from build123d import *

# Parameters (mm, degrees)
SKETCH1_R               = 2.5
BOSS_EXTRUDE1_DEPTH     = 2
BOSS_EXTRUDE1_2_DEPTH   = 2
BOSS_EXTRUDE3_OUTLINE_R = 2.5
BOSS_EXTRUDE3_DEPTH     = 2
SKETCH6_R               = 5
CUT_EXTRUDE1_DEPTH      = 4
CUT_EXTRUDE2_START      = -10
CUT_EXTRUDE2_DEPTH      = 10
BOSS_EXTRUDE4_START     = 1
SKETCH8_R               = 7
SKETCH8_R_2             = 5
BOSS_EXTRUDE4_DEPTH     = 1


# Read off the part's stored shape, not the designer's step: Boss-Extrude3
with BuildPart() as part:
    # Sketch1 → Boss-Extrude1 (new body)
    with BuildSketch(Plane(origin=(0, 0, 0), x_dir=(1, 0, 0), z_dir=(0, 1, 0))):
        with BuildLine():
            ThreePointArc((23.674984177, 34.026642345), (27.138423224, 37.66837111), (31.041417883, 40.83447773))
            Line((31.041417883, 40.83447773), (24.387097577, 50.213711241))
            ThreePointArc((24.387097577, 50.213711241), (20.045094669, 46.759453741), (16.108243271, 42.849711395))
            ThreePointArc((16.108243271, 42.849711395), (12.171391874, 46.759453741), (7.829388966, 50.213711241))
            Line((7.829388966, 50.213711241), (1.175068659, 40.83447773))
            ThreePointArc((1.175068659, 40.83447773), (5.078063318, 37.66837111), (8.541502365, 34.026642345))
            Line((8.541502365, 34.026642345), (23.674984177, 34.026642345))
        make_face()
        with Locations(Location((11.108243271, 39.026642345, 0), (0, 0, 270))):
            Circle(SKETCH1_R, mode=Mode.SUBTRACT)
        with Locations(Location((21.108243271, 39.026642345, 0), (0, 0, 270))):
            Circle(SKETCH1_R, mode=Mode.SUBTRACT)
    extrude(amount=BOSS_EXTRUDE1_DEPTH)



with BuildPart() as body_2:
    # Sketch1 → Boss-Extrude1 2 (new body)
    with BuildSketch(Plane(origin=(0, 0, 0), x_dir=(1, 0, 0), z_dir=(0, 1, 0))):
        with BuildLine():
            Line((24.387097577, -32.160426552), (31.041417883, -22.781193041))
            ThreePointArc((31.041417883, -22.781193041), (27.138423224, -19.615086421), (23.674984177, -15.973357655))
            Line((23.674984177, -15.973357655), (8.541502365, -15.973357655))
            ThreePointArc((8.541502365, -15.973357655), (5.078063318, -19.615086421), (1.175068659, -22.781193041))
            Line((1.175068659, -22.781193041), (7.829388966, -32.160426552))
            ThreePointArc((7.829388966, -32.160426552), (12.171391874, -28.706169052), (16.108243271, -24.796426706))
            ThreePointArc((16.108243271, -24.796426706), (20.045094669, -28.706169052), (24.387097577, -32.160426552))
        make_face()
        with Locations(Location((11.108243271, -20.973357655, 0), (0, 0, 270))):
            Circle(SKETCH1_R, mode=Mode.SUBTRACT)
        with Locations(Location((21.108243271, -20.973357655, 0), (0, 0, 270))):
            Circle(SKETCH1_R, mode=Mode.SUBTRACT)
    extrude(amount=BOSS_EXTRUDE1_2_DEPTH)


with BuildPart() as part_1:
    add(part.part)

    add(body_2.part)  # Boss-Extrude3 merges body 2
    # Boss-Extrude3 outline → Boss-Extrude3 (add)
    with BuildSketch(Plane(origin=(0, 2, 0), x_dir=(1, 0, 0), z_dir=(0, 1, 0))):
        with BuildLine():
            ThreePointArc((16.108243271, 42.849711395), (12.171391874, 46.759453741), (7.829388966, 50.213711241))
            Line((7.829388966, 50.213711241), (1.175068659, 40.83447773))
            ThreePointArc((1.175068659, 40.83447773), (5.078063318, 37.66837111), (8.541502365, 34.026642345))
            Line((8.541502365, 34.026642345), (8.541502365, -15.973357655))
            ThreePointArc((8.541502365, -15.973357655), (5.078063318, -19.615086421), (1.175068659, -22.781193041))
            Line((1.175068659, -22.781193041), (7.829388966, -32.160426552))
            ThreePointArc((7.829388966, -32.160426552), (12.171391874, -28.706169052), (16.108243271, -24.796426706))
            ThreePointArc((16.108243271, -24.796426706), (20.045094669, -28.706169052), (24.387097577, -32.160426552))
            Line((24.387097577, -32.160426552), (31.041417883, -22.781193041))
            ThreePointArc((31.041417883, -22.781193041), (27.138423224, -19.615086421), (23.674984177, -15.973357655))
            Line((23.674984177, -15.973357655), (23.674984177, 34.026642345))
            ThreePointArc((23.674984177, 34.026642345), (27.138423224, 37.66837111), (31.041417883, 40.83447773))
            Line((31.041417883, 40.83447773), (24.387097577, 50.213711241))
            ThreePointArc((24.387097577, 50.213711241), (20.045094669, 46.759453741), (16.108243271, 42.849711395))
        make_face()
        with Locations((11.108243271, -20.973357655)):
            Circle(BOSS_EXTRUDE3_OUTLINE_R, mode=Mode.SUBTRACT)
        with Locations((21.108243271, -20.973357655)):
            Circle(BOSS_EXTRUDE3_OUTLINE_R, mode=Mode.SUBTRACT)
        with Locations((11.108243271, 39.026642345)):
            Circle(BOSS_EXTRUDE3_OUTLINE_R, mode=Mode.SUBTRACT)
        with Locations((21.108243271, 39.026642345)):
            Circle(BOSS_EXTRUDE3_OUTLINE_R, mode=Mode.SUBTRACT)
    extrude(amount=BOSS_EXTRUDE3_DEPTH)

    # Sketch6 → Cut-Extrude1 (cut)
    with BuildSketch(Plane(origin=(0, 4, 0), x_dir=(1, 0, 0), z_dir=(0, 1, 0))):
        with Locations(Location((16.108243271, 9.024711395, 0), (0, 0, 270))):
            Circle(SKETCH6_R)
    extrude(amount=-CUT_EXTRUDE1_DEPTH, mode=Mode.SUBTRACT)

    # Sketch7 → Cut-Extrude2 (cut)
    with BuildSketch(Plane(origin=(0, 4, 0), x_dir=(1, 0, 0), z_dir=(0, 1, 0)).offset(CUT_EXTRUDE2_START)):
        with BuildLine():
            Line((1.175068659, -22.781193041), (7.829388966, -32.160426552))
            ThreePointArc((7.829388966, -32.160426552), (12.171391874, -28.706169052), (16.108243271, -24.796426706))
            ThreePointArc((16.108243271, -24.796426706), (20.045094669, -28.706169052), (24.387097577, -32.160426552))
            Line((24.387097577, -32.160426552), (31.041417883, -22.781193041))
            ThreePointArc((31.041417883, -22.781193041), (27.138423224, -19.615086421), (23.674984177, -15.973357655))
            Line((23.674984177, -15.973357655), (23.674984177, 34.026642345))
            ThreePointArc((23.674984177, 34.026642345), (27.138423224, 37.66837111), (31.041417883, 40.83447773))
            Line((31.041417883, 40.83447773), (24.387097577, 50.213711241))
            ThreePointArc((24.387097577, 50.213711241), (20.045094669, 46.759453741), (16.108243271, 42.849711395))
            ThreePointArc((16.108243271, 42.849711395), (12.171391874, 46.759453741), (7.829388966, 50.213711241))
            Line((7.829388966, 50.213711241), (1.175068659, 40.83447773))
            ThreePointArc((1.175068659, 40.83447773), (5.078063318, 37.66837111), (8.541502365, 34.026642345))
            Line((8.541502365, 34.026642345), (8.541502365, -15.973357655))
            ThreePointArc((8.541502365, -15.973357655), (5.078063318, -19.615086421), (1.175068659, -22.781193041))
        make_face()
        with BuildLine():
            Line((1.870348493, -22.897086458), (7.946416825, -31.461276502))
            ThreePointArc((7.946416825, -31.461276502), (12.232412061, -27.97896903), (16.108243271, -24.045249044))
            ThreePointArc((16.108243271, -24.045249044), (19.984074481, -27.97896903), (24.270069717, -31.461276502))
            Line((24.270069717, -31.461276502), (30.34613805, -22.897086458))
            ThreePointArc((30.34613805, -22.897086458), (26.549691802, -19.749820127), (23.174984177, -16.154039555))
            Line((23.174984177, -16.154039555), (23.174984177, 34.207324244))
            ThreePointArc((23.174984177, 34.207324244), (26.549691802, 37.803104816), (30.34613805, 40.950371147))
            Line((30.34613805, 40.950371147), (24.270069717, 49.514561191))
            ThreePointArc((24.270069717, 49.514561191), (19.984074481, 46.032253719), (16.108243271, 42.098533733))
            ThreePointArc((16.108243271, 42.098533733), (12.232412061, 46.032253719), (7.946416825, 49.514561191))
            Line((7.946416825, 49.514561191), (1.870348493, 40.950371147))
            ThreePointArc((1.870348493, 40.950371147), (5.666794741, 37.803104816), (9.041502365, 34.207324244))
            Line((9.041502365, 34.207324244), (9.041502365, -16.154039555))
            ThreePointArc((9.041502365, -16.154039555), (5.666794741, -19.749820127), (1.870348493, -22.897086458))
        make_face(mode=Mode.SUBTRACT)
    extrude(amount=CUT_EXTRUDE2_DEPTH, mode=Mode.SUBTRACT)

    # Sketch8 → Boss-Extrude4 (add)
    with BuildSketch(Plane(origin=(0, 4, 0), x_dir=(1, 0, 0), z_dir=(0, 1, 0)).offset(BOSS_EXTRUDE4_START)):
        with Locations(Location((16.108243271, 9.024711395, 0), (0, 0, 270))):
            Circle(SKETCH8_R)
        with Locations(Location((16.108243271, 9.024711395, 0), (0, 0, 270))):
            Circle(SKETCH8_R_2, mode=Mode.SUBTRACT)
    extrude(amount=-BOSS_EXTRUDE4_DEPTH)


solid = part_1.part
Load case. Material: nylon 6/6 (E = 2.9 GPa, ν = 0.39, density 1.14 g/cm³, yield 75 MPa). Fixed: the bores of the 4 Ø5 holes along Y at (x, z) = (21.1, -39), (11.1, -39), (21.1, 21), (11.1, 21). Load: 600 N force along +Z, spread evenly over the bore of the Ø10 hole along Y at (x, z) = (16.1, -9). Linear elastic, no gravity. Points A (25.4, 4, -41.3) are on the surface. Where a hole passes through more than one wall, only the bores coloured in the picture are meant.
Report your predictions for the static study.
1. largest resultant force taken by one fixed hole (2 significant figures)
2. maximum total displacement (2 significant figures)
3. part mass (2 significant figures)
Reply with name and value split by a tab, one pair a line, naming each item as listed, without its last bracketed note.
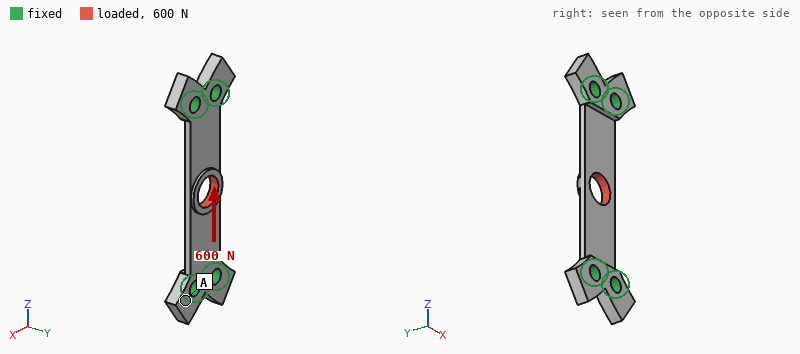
largest resultant force taken by one fixed hole	160 N
maximum total displacement	0.12 mm
part mass	3.7 g
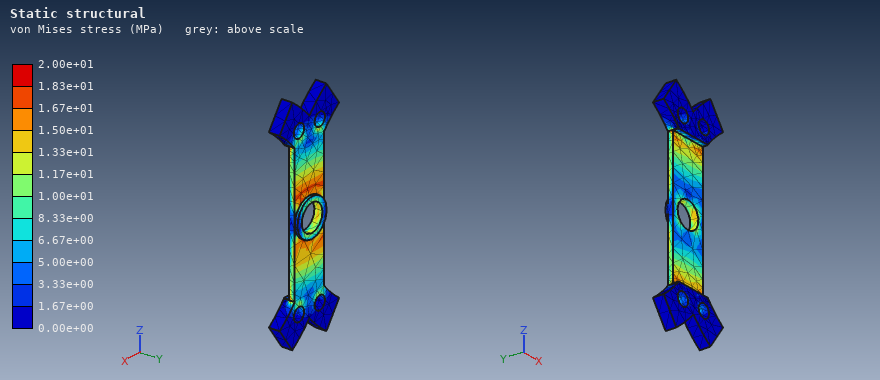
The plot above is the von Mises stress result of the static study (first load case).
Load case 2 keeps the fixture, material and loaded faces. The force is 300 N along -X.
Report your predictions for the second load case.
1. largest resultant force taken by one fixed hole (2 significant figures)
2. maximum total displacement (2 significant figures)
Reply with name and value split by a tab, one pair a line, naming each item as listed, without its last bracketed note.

largest resultant force taken by one fixed hole	210 N
maximum total displacement	0.44 mm
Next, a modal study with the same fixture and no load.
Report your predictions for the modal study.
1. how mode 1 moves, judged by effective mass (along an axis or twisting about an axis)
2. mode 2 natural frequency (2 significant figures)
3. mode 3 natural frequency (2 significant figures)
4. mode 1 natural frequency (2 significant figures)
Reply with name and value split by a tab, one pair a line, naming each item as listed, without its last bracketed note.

how mode 1 moves, judged by effective mass	along Y
mode 2 natural frequency	2800 Hz
mode 3 natural frequency	3300 Hz
mode 1 natural frequency	1300 Hz
